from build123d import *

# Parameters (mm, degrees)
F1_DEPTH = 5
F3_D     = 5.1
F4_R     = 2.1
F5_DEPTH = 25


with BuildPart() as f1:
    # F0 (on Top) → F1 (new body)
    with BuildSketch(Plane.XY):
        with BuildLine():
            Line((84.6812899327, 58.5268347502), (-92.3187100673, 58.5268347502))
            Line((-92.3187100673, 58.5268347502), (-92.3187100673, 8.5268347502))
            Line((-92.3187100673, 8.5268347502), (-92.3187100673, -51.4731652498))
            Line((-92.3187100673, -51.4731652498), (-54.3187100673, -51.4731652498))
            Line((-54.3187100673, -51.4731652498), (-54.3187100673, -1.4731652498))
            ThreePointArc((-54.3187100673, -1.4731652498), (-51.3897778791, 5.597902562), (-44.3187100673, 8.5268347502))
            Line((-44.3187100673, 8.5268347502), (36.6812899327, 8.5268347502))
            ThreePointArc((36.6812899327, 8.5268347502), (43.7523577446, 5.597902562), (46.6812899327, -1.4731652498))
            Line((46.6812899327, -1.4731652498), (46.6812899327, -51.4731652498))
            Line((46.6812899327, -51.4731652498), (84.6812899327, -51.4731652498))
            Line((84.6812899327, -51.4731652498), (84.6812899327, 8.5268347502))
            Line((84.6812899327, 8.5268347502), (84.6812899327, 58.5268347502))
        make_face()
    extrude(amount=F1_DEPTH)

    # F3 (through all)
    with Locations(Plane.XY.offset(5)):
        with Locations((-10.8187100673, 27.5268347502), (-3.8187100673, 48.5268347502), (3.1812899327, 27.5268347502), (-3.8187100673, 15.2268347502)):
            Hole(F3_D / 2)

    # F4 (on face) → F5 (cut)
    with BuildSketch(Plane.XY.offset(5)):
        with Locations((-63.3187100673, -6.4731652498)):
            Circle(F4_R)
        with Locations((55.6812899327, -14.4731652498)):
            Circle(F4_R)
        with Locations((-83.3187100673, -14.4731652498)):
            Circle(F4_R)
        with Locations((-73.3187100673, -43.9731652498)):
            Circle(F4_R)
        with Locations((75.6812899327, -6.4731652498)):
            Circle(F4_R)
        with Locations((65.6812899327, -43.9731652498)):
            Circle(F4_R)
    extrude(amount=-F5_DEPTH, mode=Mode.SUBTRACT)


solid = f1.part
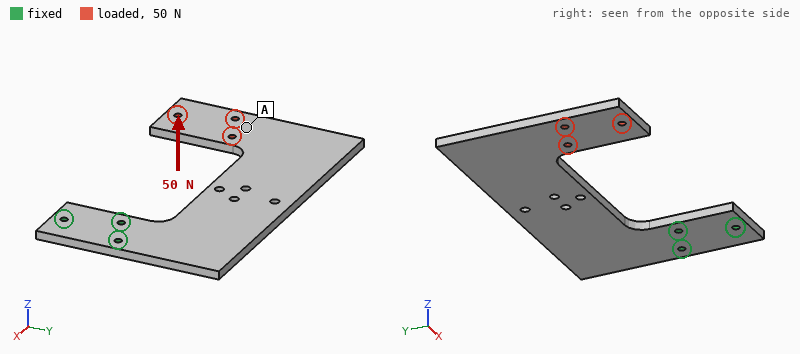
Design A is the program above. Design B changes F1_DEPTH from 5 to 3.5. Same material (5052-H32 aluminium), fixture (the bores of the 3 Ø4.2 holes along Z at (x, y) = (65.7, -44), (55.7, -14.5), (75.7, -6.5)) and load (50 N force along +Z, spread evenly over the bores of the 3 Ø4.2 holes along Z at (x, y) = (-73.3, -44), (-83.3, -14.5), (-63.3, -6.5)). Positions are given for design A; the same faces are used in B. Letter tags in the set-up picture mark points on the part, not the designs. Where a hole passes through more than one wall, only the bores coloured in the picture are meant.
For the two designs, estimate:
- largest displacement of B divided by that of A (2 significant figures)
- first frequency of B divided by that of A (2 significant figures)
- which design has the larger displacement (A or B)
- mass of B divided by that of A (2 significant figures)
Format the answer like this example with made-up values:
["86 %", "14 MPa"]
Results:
["2.9", "0.71", "B", "0.70"]
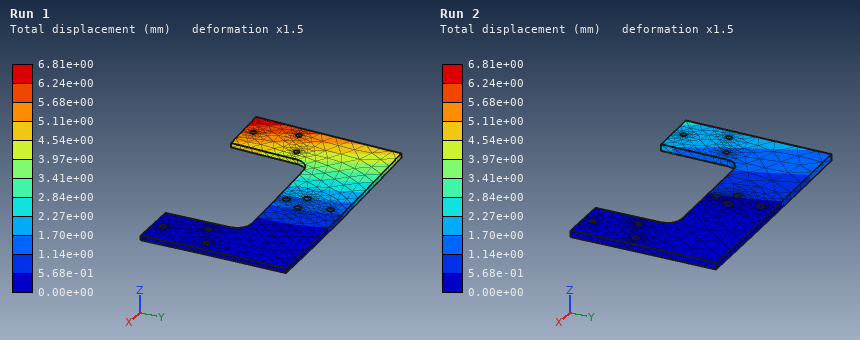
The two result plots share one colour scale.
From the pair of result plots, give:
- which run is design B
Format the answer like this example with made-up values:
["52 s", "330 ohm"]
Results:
["Run 1"]
